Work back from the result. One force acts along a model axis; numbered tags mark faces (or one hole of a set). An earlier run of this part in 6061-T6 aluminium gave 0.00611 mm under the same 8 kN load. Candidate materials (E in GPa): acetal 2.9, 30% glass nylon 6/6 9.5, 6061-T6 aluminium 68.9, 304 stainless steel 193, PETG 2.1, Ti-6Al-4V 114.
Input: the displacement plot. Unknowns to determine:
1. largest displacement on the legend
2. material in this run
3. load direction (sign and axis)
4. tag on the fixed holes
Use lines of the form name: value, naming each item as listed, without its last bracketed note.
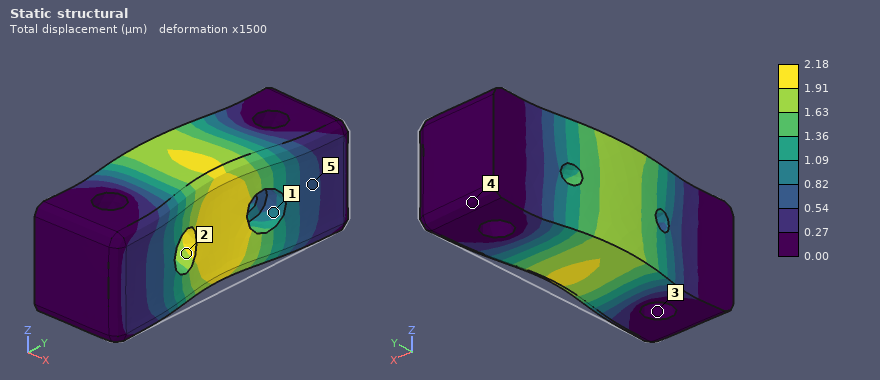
largest displacement on the legend: 2.18 µm
material in this run: 304 stainless steel
load direction: -X
tag on the fixed holes: 3
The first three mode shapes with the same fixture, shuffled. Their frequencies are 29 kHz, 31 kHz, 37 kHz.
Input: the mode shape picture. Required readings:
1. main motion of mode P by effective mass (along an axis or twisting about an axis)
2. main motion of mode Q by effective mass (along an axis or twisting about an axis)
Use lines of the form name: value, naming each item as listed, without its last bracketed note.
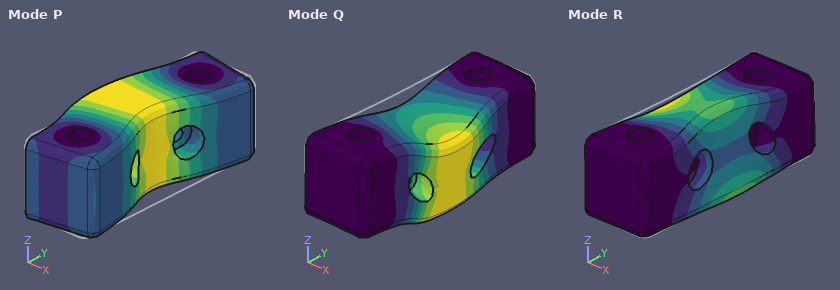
main motion of mode P by effective mass: along X
main motion of mode Q by effective mass: along Z
